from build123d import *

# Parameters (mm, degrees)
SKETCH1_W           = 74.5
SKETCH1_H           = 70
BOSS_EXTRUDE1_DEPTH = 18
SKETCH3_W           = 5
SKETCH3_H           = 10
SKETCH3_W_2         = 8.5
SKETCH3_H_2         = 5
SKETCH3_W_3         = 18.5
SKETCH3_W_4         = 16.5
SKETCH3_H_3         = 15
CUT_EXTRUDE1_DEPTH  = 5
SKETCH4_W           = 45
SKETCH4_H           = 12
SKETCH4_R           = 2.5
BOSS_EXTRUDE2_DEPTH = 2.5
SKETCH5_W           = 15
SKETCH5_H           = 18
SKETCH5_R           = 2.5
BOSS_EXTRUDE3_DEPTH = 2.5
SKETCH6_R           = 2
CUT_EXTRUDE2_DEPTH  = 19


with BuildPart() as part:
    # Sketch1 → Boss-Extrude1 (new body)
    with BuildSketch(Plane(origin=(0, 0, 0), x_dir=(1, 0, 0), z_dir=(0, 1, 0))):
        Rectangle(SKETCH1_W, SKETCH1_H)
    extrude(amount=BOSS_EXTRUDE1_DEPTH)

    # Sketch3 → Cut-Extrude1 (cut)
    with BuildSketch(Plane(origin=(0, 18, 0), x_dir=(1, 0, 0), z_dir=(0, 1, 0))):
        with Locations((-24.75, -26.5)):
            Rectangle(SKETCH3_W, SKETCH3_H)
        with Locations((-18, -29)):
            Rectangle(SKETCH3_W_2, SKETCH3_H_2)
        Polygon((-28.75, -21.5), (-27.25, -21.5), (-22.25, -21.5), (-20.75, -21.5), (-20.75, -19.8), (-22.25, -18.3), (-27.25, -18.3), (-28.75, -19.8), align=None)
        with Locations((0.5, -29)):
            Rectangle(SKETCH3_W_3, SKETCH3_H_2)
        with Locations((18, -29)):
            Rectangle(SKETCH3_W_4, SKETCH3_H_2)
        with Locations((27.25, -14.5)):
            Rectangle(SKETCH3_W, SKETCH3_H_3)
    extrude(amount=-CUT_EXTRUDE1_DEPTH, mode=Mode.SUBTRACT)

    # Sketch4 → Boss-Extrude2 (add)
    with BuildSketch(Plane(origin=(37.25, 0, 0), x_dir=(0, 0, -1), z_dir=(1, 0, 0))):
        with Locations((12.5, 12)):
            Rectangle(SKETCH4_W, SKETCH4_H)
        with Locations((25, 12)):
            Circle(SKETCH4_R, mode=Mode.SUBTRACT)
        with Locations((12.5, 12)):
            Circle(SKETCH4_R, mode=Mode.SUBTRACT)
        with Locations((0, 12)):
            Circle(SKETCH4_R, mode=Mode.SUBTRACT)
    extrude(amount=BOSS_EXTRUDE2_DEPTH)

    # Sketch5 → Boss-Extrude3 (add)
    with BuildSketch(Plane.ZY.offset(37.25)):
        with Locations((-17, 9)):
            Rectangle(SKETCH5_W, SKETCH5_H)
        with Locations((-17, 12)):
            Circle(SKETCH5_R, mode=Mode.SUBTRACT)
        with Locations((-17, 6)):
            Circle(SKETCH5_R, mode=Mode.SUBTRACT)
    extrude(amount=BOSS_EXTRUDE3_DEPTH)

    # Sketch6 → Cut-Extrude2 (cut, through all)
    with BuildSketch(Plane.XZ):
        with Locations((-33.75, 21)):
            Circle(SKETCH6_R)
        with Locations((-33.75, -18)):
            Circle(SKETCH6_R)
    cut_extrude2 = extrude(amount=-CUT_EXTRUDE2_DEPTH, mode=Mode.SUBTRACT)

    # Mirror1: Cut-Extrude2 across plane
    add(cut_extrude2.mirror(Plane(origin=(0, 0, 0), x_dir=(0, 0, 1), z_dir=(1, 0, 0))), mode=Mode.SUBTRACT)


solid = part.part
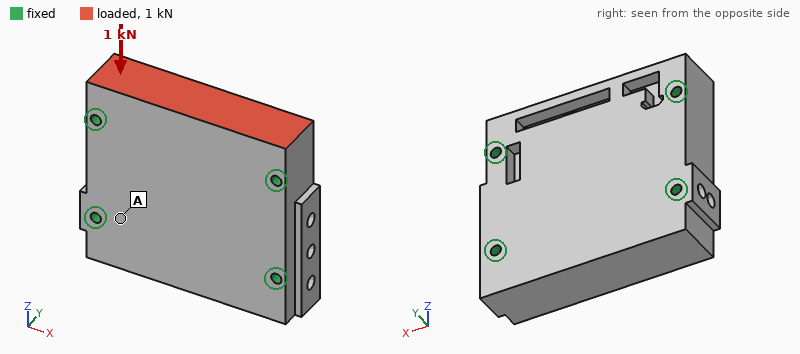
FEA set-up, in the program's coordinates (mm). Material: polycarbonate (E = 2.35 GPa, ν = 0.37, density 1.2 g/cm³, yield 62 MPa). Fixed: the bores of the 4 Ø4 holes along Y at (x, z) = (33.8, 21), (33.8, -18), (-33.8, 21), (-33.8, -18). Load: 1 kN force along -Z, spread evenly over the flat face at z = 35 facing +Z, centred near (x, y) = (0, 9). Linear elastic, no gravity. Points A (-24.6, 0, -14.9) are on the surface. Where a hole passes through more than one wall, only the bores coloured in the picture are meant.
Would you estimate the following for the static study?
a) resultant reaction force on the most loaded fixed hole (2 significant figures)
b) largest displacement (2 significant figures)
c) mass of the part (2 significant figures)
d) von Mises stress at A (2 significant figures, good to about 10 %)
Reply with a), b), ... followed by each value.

a) 330 N
b) 45 µm
c) 110 g
d) 0.54 MPa
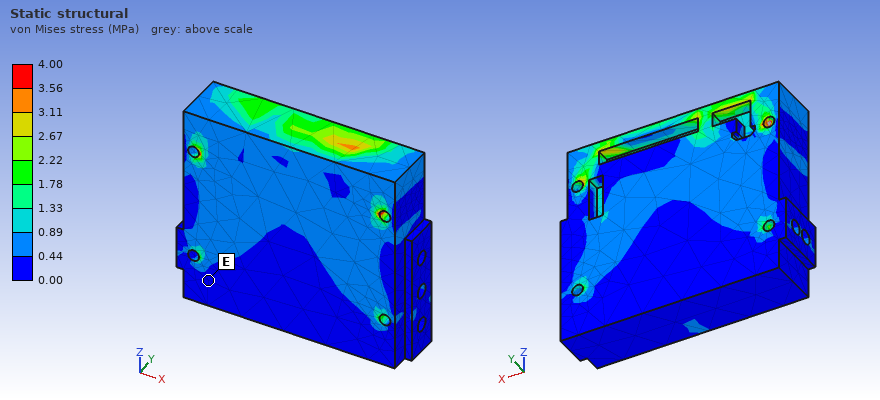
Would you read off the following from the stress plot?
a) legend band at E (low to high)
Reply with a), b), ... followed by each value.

a) 0.00 to 0.44 MPa
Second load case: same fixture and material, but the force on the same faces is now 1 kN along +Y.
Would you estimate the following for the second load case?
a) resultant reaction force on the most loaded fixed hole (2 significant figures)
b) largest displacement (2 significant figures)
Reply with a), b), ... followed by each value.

a) 560 N
b) 0.16 mm
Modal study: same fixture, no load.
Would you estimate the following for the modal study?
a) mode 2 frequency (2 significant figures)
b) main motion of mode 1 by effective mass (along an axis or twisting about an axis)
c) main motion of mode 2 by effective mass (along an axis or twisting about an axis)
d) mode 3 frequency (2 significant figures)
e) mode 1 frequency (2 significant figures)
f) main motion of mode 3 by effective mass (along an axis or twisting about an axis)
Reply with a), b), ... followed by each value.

a) 3700 Hz
b) along Y
c) twisting about X
d) 4800 Hz
e) 3100 Hz
f) along Z
